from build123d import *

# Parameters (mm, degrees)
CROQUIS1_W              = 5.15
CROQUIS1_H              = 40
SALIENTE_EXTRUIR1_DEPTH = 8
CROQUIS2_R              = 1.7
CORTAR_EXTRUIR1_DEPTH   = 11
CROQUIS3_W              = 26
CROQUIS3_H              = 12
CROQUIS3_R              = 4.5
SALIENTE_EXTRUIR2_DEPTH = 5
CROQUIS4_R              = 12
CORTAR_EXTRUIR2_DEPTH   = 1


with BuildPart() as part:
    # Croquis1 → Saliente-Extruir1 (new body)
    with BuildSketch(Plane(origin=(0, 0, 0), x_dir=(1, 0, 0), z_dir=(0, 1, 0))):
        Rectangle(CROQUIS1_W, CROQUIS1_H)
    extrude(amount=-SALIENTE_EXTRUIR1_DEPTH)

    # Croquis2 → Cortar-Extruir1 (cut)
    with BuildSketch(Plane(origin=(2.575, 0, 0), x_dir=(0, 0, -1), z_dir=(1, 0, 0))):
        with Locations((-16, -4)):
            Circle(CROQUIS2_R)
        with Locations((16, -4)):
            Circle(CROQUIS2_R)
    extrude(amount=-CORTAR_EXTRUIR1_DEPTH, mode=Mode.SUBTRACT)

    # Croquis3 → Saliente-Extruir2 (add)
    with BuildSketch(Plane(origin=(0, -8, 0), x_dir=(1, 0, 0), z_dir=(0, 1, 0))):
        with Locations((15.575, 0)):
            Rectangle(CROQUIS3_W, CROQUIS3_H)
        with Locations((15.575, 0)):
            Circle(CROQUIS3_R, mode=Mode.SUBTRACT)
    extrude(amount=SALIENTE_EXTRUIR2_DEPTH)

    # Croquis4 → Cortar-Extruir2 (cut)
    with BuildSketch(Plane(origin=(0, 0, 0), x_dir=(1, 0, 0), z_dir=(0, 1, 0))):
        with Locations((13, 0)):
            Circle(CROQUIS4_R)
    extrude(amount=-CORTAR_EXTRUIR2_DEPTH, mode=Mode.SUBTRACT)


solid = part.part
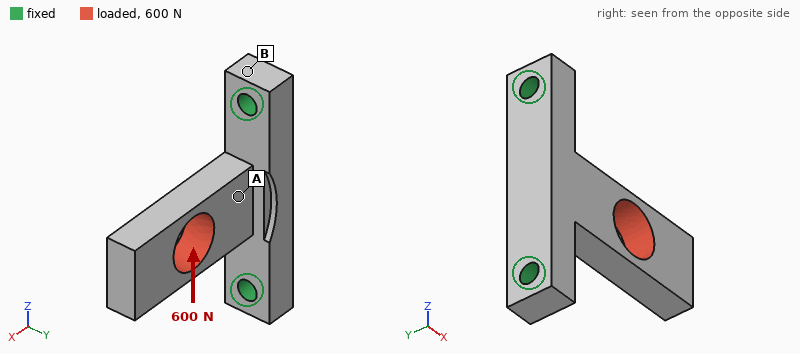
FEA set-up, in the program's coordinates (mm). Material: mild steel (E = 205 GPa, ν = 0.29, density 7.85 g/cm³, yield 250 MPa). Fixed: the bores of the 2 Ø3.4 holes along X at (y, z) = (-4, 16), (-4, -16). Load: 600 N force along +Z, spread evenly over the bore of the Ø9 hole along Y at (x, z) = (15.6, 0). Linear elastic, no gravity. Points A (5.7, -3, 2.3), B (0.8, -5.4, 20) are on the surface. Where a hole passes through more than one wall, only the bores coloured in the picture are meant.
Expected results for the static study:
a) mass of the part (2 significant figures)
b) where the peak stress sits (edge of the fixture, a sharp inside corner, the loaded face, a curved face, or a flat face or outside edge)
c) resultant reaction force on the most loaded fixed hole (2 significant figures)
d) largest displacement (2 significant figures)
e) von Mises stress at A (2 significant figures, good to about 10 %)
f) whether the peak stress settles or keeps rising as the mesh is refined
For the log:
22 g
a sharp inside corner
520 N
37 µm
32 MPa
keeps rising
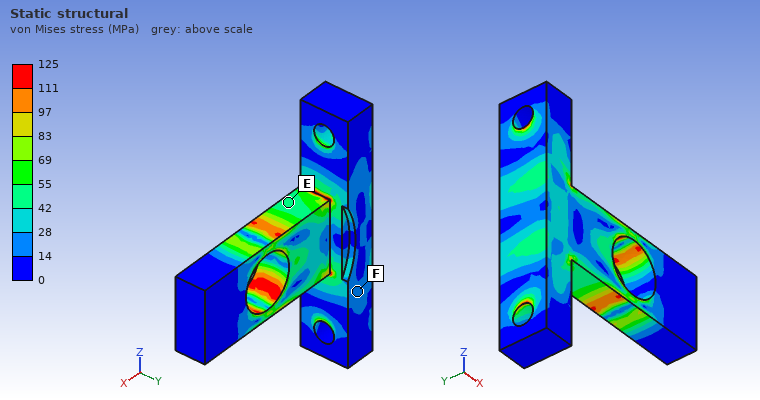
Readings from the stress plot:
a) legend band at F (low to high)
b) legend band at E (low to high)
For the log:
14 to 28 MPa
42 to 55 MPa
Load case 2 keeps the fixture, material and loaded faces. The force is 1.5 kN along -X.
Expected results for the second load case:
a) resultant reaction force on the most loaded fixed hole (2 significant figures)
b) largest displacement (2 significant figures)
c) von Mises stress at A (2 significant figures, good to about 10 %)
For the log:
770 N
24 µm
22 MPa
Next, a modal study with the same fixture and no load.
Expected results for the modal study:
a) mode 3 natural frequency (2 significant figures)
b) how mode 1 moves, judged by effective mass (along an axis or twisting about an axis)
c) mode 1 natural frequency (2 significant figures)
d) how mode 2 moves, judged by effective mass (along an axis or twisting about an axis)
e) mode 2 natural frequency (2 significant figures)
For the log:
15 kHz
along Y
3500 Hz
along Z
7300 Hz
